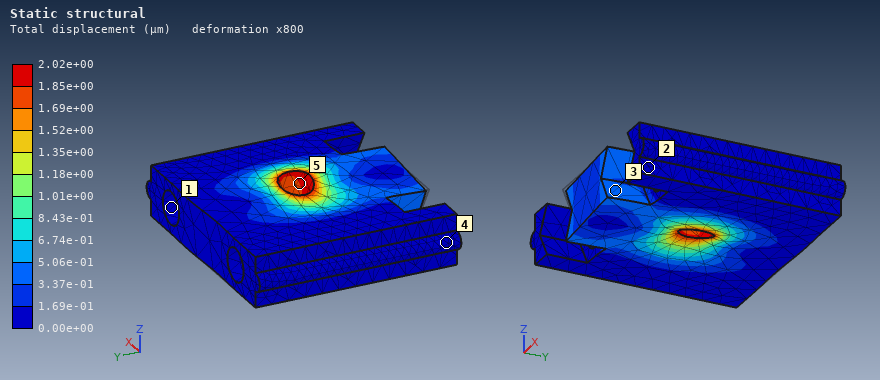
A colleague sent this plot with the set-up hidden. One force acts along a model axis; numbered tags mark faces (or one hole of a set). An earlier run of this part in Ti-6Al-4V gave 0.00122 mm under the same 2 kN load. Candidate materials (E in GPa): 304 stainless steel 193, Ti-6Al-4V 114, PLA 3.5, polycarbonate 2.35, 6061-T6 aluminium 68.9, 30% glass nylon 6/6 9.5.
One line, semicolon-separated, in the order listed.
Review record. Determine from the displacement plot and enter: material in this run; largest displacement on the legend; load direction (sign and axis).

6061-T6 aluminium; 2.02e+00 µm; +X
